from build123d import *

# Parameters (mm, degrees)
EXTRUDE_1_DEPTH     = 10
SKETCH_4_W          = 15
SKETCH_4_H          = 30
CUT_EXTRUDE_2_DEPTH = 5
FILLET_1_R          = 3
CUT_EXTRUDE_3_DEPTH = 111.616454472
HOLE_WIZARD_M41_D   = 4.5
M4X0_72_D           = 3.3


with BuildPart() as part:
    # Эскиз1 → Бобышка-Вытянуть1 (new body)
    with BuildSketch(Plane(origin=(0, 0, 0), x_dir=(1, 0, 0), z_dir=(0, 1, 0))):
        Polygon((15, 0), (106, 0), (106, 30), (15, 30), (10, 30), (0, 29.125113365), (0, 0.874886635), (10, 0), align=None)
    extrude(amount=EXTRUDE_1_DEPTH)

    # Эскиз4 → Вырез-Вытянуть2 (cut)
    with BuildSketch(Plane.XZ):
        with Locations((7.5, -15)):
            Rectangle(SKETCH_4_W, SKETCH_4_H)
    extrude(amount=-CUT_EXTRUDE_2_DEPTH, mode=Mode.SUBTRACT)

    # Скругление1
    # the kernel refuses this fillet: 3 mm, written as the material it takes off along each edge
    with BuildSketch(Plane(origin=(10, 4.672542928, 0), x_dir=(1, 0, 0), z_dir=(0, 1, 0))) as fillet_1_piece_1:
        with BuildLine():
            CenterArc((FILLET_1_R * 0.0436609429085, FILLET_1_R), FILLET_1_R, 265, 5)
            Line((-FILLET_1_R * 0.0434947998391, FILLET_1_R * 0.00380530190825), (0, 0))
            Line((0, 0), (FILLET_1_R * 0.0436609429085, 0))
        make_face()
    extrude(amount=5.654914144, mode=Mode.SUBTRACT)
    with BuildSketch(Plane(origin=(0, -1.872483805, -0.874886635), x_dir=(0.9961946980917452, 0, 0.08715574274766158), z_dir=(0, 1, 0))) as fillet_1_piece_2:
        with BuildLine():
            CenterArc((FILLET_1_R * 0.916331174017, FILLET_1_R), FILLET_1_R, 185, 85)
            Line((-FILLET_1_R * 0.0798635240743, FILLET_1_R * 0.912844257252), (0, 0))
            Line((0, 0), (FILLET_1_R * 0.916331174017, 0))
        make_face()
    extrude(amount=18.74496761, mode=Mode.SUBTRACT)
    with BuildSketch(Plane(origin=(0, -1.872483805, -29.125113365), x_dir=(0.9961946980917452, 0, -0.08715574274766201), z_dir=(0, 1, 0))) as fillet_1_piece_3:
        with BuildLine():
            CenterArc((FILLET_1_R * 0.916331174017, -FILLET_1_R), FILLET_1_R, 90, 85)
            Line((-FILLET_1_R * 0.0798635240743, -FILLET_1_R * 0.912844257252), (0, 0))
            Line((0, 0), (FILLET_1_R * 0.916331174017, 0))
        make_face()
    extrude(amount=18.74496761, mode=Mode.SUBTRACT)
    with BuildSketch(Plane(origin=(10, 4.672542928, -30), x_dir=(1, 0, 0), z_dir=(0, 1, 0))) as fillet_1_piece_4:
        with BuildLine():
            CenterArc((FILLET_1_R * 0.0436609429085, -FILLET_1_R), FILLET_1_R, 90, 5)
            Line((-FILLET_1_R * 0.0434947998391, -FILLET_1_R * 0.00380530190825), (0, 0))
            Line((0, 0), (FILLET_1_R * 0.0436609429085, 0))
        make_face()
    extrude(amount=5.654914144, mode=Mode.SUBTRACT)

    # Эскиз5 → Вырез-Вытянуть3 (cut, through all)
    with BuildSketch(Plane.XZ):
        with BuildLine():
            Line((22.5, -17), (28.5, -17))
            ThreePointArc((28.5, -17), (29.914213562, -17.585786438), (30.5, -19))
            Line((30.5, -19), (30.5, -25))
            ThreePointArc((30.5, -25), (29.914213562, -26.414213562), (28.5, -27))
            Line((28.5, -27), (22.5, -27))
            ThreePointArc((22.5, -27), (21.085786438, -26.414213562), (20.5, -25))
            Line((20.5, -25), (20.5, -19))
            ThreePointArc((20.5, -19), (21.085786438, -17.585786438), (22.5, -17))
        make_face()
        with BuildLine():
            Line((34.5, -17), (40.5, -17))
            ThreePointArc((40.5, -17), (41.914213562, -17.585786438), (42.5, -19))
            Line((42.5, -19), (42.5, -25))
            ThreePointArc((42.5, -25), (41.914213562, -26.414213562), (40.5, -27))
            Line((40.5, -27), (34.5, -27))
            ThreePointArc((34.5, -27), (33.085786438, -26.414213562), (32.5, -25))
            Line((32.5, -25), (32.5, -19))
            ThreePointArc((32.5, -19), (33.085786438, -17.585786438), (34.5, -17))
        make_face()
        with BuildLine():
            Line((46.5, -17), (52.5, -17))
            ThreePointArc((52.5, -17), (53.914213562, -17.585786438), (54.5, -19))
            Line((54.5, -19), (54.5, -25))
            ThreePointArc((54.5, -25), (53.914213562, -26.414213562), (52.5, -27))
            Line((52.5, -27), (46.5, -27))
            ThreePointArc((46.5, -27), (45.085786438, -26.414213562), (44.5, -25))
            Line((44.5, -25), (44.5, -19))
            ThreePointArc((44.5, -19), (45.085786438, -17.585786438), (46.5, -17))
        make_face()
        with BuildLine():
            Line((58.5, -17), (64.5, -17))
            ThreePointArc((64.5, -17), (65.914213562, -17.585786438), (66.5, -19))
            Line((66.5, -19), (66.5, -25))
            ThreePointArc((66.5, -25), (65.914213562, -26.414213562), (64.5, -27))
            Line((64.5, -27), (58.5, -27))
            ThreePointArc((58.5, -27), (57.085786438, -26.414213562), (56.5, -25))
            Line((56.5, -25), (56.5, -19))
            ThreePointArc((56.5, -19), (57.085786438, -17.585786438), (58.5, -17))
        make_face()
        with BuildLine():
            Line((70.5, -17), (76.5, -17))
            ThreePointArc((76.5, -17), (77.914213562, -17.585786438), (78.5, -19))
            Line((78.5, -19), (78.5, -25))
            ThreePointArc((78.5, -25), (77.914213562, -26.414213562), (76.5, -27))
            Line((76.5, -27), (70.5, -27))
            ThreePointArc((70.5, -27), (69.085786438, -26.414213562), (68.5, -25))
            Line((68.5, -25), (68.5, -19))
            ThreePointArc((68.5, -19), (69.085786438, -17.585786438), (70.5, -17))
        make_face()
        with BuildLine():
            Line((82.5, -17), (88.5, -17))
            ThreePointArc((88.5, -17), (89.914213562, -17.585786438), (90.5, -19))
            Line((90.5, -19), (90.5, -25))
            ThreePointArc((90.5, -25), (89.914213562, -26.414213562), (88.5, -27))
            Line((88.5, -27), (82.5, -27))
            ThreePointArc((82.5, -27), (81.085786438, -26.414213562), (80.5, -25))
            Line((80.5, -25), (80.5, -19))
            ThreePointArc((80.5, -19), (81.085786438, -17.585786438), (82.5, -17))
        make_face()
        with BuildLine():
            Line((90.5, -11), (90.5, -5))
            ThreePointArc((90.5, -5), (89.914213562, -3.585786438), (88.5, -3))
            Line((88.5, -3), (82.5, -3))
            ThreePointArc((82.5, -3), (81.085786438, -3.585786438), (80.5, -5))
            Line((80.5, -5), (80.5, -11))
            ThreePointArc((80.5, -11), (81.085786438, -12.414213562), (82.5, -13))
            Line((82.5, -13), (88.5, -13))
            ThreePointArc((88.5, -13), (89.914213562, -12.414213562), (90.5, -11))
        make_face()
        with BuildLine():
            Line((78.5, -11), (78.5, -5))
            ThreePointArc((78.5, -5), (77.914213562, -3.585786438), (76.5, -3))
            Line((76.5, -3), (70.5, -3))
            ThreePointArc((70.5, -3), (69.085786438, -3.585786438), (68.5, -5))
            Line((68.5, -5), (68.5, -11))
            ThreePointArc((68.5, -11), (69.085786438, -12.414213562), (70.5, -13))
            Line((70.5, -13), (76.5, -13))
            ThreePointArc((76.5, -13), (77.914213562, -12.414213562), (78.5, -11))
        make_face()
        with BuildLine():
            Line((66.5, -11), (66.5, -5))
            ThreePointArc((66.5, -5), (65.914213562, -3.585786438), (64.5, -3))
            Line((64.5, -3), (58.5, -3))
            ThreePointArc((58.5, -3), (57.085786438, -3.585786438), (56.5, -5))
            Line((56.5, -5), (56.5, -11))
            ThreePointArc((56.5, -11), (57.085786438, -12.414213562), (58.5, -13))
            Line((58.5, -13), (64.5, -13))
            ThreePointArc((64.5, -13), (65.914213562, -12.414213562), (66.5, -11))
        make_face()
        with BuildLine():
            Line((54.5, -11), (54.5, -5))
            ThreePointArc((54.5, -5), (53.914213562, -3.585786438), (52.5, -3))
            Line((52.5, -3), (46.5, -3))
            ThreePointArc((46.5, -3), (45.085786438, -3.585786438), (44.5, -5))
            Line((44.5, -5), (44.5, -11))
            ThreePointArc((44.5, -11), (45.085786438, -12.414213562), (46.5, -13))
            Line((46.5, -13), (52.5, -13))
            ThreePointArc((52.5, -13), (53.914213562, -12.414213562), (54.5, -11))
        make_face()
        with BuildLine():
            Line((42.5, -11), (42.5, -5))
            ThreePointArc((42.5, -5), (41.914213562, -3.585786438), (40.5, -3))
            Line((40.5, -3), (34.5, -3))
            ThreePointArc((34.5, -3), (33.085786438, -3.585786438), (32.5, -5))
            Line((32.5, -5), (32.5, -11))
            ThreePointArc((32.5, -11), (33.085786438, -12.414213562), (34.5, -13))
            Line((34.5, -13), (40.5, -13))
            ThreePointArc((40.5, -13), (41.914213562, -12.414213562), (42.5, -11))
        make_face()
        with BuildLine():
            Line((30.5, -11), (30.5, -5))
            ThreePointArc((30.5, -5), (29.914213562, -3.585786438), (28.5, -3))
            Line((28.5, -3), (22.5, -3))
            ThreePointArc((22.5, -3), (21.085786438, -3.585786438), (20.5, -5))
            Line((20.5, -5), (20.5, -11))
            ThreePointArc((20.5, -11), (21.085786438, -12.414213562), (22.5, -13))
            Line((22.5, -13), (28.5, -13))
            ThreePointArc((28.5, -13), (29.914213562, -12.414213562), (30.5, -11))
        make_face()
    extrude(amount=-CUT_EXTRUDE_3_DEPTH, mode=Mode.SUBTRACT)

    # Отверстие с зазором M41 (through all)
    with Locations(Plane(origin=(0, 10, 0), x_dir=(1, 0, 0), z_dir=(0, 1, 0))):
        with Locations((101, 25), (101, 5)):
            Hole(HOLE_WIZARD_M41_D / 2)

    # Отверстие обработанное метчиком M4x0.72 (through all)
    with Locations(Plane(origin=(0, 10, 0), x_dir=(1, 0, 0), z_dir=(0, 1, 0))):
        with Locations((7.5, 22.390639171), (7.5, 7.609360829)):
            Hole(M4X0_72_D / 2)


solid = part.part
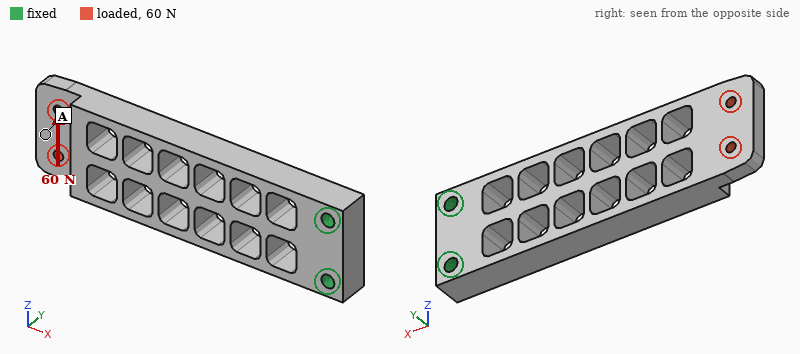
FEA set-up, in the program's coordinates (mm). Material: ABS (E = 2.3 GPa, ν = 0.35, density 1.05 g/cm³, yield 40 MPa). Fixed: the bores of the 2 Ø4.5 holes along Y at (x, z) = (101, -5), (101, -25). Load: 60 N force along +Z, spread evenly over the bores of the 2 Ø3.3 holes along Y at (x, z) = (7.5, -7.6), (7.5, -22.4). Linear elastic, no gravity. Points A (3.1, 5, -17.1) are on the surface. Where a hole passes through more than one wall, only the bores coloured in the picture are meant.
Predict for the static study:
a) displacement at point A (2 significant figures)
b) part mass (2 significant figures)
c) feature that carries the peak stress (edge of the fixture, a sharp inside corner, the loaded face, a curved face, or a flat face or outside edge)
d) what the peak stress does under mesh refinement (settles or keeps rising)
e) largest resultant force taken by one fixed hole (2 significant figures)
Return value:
1.2 mm
18 g
a sharp inside corner
keeps rising
250 N
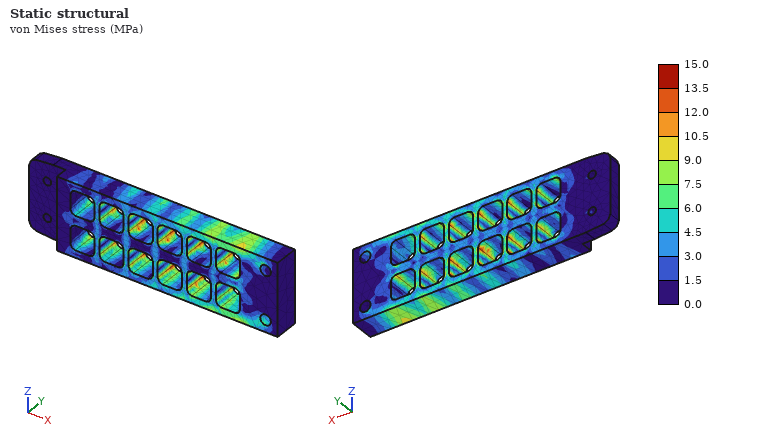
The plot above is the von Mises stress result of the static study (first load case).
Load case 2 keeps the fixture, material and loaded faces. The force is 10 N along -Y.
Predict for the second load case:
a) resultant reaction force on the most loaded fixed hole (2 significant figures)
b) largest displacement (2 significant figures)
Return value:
5.0 N
1.3 mm
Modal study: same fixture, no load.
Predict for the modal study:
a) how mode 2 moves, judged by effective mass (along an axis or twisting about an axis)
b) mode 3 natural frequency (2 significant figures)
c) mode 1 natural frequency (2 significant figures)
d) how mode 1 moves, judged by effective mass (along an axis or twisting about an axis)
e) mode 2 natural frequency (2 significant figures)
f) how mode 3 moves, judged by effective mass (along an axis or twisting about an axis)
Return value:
along Z
680 Hz
210 Hz
along Y
460 Hz
twisting about X
